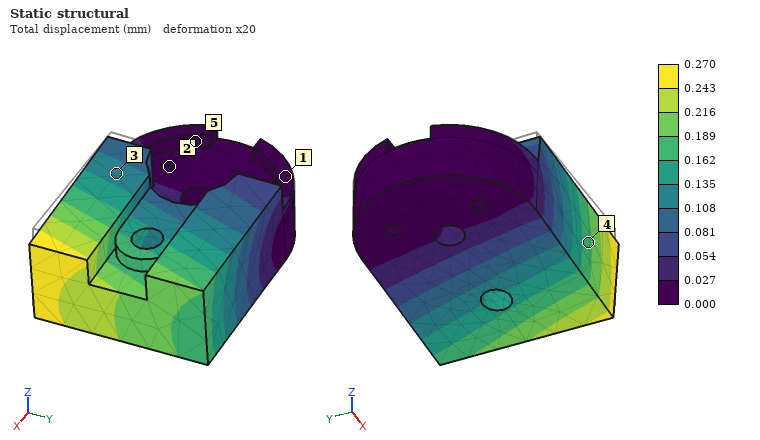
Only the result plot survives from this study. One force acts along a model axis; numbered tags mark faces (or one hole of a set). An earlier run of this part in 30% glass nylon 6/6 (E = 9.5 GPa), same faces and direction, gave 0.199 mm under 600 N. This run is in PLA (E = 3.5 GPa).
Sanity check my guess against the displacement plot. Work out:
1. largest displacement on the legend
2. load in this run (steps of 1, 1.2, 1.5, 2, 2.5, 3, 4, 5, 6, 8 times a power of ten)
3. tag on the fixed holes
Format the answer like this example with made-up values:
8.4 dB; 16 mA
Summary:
0.270 mm; 300 N; 2
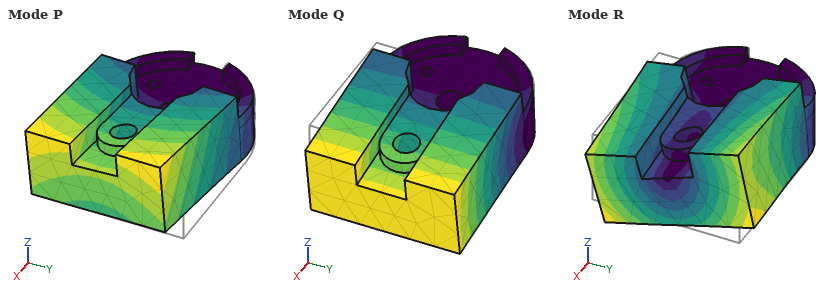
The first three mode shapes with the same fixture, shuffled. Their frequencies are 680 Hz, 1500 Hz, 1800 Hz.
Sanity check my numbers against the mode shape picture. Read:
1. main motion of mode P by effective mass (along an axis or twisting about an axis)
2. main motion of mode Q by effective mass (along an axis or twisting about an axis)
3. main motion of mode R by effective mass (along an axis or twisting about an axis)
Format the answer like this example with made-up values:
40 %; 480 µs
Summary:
along Y; along Z; twisting about X
